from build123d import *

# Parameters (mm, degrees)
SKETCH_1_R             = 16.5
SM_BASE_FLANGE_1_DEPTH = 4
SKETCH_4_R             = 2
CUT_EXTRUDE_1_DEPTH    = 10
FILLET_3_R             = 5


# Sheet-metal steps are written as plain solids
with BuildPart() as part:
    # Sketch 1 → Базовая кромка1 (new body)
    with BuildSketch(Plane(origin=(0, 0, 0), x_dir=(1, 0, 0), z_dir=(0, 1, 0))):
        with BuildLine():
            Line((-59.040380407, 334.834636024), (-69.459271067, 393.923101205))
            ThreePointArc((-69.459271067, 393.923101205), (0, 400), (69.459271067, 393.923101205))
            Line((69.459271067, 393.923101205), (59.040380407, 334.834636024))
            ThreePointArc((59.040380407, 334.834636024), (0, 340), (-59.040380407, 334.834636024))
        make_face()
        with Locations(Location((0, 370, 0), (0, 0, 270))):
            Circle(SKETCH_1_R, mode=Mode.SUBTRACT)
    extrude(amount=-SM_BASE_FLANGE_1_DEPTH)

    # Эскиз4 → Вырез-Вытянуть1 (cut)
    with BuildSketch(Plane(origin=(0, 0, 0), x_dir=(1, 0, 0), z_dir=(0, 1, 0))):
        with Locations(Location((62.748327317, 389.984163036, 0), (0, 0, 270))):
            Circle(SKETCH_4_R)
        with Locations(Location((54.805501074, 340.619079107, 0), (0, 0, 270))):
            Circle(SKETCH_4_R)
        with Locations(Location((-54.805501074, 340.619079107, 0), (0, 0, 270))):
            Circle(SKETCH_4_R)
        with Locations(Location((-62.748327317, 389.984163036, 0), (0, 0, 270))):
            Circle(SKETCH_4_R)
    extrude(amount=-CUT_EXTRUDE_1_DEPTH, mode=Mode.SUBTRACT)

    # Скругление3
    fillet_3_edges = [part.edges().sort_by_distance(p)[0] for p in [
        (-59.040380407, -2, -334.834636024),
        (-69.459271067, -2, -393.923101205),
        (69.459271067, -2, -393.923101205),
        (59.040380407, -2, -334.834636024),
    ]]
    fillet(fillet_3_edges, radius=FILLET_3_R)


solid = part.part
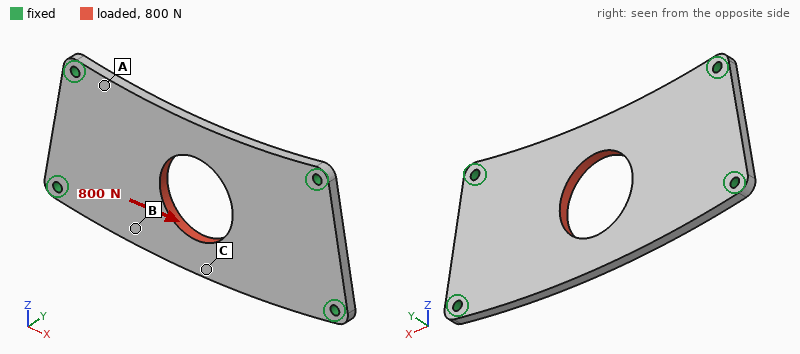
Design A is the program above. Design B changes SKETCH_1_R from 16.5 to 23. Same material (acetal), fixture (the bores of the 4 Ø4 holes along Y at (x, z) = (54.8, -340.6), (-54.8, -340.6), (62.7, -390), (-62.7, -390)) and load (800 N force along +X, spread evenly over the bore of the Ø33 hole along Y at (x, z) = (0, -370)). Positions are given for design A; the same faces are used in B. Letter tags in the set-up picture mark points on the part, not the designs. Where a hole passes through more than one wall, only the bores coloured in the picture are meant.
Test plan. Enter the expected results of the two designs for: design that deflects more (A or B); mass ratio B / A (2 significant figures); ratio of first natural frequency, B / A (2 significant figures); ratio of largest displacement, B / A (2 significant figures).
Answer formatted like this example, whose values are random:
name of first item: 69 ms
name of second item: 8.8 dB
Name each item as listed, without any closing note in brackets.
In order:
design that deflects more: B
mass ratio B / A: 0.88
ratio of first natural frequency, B / A: 1.1
ratio of largest displacement, B / A: 1.1
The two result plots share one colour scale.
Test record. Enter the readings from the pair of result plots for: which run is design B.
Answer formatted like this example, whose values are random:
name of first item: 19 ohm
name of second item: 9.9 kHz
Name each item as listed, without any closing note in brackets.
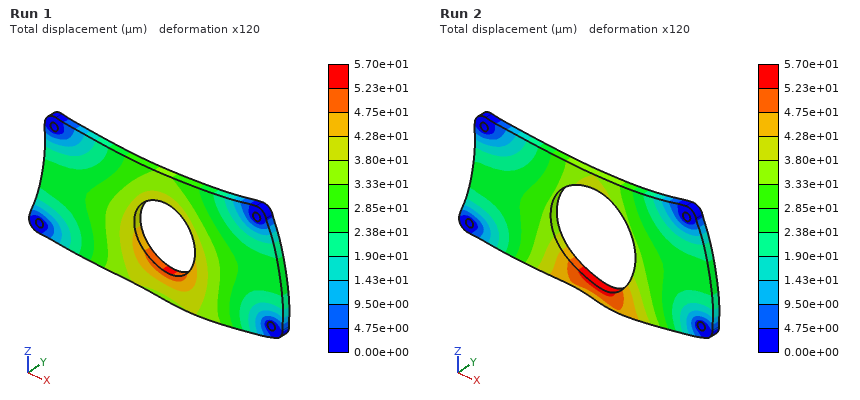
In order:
which run is design B: Run 2
